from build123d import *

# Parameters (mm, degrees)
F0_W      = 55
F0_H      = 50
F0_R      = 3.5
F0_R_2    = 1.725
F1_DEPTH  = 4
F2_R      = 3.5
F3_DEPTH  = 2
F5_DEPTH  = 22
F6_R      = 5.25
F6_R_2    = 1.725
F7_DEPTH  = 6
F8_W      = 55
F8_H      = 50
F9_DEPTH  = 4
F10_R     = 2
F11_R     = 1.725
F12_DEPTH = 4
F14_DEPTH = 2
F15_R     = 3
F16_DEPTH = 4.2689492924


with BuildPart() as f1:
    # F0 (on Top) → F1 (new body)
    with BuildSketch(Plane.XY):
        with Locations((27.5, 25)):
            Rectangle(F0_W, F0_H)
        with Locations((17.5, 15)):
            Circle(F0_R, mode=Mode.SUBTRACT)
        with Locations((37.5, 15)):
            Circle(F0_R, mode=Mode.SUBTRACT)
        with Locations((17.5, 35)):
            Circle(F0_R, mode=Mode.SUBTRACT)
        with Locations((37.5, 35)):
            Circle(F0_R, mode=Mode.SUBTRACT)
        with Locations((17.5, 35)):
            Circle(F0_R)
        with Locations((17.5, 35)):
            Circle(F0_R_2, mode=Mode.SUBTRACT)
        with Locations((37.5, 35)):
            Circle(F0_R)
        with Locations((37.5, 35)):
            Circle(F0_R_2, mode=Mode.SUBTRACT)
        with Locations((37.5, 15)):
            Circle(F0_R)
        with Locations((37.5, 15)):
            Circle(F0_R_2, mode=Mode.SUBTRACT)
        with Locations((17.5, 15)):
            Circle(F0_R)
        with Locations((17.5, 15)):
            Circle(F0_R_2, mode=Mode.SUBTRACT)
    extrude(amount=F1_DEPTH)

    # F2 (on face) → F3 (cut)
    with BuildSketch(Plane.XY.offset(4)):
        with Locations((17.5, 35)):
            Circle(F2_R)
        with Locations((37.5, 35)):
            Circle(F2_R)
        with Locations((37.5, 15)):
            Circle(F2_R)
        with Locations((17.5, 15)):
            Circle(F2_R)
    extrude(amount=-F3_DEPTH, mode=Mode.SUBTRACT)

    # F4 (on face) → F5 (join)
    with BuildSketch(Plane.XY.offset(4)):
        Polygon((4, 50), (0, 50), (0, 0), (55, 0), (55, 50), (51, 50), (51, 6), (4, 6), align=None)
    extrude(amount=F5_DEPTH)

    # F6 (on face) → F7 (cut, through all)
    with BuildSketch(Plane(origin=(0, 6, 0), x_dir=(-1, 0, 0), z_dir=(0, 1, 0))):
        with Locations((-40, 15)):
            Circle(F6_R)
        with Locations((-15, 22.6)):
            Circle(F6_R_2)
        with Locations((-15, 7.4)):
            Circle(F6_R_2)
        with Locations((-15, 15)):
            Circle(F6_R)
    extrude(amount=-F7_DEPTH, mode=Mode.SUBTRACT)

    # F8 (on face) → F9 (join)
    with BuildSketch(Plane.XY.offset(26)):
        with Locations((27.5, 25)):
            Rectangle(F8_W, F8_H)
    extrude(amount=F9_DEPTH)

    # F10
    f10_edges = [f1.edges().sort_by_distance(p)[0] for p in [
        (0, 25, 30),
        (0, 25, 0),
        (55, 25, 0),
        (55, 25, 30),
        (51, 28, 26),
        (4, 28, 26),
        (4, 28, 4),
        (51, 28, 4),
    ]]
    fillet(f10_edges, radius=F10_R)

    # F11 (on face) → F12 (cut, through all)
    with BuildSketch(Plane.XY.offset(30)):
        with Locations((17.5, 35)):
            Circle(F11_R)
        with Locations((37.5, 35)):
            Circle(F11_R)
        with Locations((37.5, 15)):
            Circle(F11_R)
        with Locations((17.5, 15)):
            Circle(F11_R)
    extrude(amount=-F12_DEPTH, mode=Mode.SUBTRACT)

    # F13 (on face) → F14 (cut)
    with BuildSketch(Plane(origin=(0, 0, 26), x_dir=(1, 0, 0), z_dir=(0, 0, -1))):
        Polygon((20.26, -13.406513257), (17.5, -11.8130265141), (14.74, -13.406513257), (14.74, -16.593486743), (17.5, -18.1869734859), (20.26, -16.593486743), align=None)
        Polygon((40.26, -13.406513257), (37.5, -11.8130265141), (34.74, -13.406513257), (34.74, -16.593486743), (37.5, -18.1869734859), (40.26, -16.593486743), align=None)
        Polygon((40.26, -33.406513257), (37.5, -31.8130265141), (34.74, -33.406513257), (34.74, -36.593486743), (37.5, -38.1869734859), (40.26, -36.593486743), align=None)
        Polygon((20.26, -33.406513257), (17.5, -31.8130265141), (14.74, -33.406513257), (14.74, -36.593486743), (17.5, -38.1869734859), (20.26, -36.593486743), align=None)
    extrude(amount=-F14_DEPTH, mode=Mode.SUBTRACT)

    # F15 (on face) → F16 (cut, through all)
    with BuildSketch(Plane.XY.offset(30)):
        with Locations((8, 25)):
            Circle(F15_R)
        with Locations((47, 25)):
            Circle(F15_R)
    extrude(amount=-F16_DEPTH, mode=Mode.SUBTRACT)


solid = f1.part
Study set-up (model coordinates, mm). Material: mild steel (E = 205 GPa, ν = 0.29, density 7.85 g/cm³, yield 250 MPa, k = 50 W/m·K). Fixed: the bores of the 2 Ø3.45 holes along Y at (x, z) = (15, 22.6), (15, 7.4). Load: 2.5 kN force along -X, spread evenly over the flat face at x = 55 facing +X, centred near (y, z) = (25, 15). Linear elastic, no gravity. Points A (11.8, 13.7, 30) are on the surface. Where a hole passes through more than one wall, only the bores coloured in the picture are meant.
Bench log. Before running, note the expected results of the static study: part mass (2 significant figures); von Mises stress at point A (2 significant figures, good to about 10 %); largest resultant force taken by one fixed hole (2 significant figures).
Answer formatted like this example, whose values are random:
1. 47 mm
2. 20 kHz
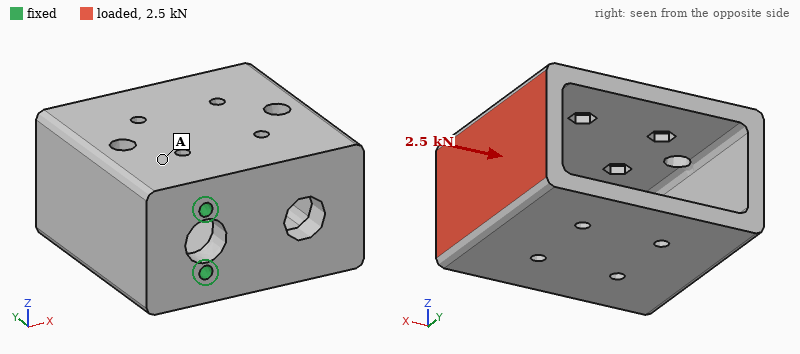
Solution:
1. 270 g
2. 31 MPa
3. 1.3 kN
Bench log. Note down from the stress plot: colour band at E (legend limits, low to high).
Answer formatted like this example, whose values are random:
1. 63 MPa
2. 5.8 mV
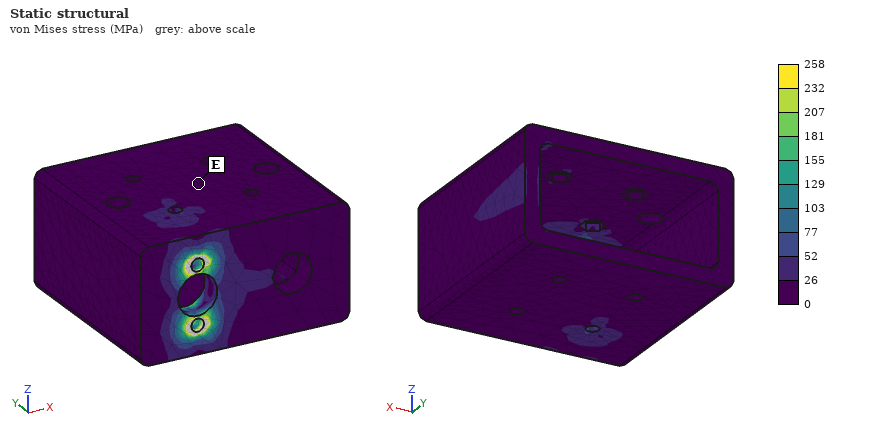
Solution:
1. 0 to 26 MPa
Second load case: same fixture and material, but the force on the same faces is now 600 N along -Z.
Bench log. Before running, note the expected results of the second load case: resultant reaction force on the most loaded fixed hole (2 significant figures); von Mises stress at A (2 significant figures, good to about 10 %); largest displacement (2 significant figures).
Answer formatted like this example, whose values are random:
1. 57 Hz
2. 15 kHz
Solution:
1. 1.5 kN
2. 6.2 MPa
3. 26 µm
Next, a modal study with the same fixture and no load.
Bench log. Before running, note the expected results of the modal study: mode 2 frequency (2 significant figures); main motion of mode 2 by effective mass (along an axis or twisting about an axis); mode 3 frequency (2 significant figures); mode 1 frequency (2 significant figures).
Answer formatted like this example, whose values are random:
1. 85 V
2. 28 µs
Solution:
1. 2700 Hz
2. along Z
3. 4900 Hz
4. 1600 Hz
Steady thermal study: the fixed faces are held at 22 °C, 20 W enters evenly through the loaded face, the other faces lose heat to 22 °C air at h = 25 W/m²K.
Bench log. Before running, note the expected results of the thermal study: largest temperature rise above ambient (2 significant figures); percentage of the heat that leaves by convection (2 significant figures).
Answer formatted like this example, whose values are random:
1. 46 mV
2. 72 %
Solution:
1. 42 K
2. 39 %
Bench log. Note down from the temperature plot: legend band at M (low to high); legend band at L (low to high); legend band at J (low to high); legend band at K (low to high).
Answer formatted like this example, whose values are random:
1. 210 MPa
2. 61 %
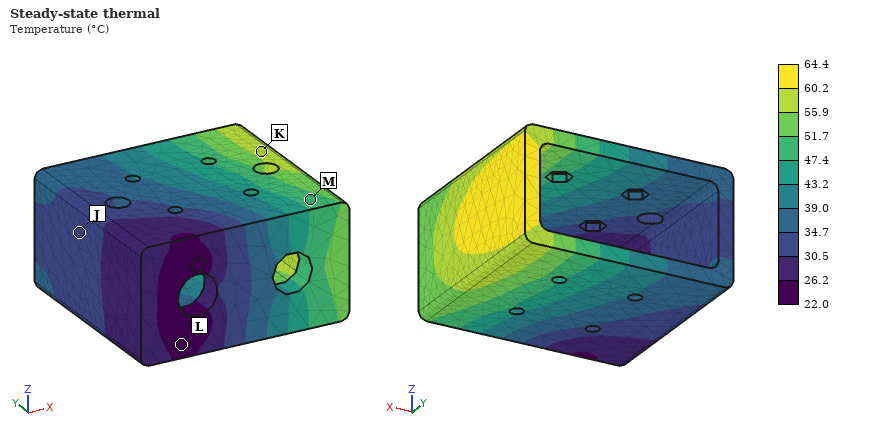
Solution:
1. 47.4 to 51.7 °C
2. 22.0 to 26.2 °C
3. 30.5 to 34.7 °C
4. 55.9 to 60.2 °C
